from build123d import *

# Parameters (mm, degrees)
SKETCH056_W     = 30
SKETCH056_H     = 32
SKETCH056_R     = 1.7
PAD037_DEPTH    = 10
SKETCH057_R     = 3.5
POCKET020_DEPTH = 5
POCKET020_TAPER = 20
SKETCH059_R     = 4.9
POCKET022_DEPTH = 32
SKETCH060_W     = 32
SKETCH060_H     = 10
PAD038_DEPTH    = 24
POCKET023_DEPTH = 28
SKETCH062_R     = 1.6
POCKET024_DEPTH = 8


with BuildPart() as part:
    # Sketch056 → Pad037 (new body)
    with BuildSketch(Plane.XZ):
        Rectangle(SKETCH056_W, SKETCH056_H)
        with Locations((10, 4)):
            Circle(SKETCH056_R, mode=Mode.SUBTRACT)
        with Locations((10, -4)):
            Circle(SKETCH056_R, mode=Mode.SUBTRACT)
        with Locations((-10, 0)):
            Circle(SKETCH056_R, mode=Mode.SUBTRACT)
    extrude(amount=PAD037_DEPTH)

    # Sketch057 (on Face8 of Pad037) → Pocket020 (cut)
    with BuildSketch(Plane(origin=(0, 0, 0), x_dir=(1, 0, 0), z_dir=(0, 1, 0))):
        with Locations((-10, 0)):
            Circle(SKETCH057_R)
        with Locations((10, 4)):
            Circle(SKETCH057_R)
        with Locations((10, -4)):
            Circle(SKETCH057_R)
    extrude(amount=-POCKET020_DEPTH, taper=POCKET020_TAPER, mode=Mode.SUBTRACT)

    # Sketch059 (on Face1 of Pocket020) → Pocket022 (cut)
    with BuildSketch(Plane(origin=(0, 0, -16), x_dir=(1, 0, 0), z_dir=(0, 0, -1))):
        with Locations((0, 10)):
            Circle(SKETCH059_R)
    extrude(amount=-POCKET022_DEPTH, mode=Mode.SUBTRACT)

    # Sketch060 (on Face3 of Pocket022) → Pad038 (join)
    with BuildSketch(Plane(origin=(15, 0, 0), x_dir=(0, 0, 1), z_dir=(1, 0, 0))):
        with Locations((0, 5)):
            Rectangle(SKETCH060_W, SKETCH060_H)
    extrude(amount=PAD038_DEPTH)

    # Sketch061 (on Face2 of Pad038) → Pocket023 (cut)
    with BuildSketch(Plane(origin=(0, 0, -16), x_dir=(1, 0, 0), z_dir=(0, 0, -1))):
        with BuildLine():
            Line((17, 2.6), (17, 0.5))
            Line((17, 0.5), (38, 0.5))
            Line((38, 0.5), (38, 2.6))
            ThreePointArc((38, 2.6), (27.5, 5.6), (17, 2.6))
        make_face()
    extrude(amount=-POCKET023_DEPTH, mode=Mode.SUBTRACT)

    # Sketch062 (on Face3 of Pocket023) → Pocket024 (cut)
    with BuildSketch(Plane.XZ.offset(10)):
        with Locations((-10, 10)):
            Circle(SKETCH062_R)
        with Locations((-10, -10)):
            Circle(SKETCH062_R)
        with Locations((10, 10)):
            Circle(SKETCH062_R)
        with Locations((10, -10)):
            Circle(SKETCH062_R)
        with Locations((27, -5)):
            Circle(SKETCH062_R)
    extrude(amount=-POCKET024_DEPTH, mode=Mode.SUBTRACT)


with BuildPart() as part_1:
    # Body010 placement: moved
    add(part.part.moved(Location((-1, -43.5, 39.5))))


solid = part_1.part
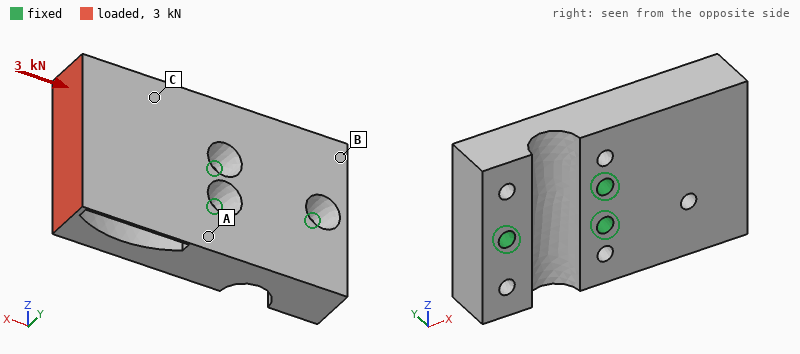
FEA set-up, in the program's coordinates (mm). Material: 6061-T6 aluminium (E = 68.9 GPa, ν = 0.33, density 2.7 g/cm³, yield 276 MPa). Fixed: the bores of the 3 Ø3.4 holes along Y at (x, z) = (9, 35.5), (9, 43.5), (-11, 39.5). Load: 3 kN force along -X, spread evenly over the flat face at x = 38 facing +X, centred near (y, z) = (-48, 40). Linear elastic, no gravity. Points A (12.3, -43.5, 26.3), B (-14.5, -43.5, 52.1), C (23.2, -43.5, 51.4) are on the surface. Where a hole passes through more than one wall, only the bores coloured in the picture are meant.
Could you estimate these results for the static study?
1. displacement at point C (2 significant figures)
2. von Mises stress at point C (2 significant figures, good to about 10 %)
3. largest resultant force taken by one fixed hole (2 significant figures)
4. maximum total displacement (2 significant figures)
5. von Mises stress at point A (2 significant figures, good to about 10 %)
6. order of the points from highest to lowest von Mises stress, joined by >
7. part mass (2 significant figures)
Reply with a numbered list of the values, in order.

1. 10 µm
2. 29 MPa
3. 1.3 kN
4. 35 µm
5. 12 MPa
6. C > A > B
7. 35 g
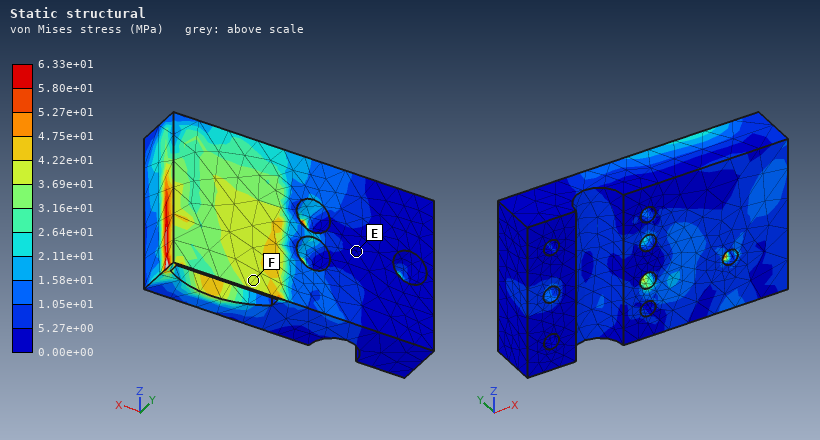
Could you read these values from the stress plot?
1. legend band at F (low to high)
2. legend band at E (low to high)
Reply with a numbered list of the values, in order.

1. 3.69e+01 to 4.22e+01 MPa
2. 0.00e+00 to 5.27e+00 MPa
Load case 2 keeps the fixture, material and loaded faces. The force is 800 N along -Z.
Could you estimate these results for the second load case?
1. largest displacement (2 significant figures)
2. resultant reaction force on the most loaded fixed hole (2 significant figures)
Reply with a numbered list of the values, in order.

1. 28 µm
2. 1.3 kN
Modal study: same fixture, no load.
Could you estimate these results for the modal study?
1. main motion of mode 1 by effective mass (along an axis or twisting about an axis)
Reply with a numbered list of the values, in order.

1. along Y
